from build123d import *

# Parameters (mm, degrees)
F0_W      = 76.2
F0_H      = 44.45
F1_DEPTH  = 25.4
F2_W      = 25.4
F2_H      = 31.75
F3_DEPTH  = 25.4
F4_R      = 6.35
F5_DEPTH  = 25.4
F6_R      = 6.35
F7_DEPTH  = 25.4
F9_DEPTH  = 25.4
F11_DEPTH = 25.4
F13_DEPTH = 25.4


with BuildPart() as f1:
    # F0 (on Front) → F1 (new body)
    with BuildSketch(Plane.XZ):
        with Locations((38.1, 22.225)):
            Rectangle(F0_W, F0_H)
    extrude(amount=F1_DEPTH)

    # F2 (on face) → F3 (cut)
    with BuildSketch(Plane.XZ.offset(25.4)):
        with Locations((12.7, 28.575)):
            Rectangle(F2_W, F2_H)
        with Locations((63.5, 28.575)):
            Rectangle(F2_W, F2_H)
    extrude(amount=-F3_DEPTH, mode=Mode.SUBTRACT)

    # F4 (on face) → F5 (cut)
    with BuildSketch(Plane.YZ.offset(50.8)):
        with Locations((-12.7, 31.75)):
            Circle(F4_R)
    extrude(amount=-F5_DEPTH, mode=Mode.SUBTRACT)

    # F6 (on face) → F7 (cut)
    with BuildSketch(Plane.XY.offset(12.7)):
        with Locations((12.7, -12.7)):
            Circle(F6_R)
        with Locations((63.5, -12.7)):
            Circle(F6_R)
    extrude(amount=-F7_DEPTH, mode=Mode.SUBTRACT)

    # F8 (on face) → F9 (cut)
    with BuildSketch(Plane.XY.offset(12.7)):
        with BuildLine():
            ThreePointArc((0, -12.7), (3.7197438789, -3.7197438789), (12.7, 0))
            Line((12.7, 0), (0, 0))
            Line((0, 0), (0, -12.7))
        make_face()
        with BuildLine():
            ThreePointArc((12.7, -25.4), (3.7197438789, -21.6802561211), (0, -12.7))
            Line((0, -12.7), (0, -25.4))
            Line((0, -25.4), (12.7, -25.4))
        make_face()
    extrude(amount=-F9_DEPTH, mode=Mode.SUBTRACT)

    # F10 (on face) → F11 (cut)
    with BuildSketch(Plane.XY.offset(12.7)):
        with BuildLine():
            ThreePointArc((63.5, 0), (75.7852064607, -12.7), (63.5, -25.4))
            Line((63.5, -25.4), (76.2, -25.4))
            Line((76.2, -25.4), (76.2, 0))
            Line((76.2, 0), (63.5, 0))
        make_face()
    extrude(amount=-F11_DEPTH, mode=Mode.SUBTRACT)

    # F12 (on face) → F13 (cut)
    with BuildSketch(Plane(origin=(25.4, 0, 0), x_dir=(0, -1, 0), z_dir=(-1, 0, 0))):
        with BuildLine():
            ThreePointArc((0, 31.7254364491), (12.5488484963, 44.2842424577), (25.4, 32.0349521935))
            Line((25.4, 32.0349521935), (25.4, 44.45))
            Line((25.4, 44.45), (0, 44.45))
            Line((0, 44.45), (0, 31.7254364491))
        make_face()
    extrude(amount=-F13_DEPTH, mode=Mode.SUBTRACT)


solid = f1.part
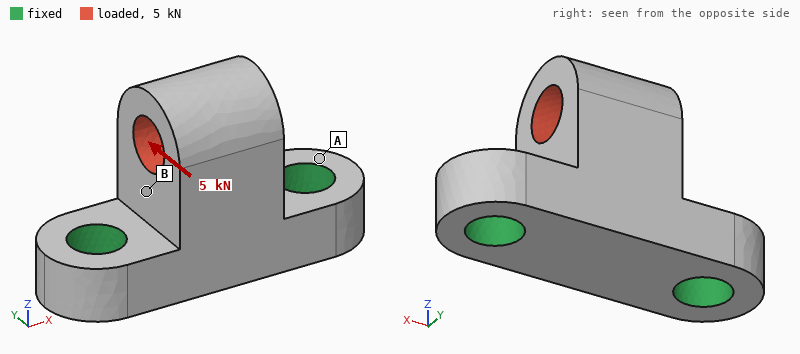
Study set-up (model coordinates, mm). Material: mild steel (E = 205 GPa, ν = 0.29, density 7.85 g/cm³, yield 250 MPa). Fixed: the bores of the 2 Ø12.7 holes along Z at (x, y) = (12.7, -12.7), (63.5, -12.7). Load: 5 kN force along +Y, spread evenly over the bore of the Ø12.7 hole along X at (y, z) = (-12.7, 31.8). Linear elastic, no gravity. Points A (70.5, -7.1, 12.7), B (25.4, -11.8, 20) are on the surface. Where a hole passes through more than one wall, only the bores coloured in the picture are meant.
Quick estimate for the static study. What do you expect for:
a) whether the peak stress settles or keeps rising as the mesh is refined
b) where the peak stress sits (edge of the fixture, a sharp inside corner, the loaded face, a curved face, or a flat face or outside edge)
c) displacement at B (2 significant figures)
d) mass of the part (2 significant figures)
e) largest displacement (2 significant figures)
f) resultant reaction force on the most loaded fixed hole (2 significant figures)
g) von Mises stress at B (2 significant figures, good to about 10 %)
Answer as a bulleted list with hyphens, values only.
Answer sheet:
- keeps rising
- edge of the fixture
- 12 µm
- 270 g
- 36 µm
- 2.5 kN
- 38 MPa
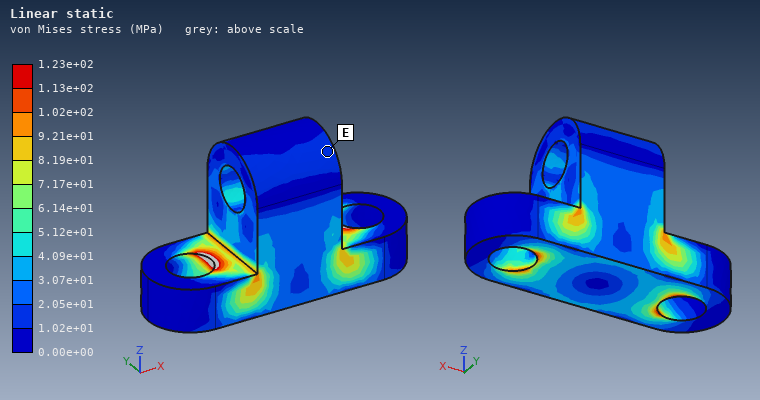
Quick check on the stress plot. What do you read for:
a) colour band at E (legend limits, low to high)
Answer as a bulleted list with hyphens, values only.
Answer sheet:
- 1.02e+01 to 2.05e+01 MPa
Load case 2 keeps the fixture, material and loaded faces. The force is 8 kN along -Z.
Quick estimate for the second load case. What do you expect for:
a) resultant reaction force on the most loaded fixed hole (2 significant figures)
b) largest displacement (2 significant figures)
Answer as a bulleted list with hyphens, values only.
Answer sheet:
- 4.2 kN
- 6.2 µm
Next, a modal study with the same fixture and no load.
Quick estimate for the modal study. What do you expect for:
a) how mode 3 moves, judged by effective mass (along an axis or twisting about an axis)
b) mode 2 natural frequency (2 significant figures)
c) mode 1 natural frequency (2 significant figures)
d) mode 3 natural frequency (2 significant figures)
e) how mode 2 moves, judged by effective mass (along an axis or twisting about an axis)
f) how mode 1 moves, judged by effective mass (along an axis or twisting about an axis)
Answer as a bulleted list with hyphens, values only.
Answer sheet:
- along Z
- 12 kHz
- 7100 Hz
- 17 kHz
- along X
- along Y
